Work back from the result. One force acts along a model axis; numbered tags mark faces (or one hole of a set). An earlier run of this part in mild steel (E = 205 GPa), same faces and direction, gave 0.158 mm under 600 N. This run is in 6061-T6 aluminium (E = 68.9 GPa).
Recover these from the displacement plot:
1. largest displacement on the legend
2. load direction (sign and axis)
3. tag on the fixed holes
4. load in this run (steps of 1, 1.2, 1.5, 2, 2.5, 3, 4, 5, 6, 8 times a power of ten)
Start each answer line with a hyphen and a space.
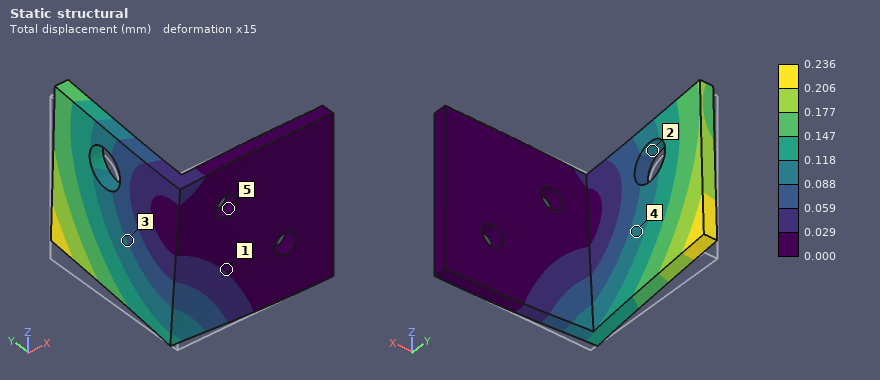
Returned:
- 0.236 mm
- +Z
- 5
- 300 N
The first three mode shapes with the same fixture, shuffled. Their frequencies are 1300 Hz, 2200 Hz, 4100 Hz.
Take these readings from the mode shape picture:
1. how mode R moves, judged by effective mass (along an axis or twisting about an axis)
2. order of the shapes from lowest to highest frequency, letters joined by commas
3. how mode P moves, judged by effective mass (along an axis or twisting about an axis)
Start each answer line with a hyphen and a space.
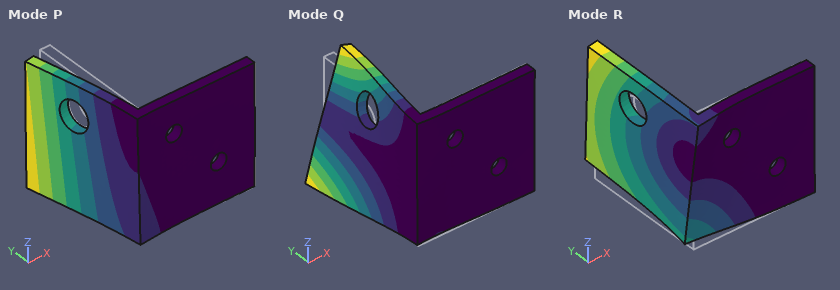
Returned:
- along Z
- P, R, Q
- along X
